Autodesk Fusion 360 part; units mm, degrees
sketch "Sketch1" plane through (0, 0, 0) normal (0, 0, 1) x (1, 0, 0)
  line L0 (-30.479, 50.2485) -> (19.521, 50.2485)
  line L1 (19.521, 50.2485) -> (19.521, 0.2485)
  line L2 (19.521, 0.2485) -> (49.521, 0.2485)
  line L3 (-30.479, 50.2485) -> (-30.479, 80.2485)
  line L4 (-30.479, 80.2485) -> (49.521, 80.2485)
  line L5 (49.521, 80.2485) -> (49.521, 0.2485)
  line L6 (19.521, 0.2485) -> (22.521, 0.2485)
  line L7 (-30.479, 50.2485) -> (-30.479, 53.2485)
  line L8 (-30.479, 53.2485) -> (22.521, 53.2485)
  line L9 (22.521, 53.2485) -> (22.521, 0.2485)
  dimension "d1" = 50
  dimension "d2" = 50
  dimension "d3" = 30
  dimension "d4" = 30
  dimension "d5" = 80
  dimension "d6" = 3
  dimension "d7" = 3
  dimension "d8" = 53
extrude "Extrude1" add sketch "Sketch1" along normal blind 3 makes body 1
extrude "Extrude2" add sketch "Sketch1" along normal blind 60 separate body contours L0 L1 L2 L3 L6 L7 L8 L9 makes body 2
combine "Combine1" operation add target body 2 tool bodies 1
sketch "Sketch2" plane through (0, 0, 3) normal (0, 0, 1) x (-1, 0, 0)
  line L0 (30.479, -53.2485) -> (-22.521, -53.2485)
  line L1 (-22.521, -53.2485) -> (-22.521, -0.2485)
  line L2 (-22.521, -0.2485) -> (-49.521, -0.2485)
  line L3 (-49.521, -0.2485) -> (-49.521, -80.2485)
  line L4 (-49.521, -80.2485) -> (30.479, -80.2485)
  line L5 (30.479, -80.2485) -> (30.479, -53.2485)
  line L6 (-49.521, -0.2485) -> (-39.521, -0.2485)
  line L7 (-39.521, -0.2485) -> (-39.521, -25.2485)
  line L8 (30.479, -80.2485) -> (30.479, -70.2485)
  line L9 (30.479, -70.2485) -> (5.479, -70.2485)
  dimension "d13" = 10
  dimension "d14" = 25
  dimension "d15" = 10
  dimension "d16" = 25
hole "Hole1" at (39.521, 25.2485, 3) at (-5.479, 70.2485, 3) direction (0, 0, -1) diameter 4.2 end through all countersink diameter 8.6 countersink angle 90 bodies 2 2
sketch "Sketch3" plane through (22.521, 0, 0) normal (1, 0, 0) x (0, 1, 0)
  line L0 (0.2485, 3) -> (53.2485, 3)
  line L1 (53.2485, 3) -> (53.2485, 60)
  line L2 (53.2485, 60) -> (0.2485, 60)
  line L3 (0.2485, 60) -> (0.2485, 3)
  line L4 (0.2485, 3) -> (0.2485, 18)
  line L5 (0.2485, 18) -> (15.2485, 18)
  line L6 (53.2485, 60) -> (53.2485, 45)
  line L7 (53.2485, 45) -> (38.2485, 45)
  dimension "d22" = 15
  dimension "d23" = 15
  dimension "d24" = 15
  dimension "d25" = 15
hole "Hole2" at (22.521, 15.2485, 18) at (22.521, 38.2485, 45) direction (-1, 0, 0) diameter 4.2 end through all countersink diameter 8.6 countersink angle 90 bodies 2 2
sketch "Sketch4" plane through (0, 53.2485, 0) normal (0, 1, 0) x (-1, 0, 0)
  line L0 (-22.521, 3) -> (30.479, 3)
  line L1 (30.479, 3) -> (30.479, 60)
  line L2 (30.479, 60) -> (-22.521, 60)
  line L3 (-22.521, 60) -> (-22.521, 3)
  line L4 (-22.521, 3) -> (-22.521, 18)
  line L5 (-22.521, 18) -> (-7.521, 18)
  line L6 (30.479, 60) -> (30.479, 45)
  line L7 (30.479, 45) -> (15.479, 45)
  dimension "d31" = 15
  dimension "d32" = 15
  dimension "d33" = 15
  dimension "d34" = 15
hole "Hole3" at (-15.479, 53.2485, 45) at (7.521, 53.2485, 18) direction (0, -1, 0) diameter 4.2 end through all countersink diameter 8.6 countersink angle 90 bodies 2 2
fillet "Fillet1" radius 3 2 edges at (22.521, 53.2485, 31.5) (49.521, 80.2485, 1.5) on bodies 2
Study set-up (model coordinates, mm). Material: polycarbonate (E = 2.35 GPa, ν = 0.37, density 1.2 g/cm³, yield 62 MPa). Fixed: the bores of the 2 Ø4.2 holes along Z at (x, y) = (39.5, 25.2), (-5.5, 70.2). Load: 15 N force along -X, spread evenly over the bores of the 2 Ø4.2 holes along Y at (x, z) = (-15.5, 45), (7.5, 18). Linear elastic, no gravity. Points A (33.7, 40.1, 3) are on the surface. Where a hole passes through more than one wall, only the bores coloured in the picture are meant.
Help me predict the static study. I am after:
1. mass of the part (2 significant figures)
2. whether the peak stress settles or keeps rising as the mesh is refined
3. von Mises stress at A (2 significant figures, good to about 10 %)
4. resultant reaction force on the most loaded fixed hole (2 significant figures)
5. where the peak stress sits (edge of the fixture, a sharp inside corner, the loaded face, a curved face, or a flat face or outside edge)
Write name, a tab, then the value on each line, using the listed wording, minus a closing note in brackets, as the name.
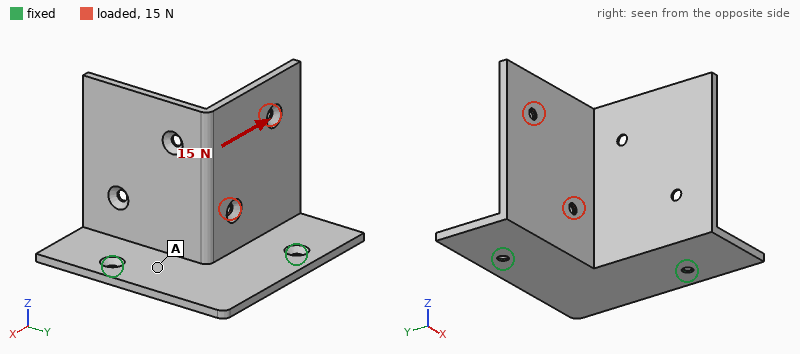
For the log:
mass of the part	34 g
whether the peak stress settles or keeps rising as the mesh is refined	keeps rising
von Mises stress at A	1.2 MPa
resultant reaction force on the most loaded fixed hole	9.9 N
where the peak stress sits	edge of the fixture
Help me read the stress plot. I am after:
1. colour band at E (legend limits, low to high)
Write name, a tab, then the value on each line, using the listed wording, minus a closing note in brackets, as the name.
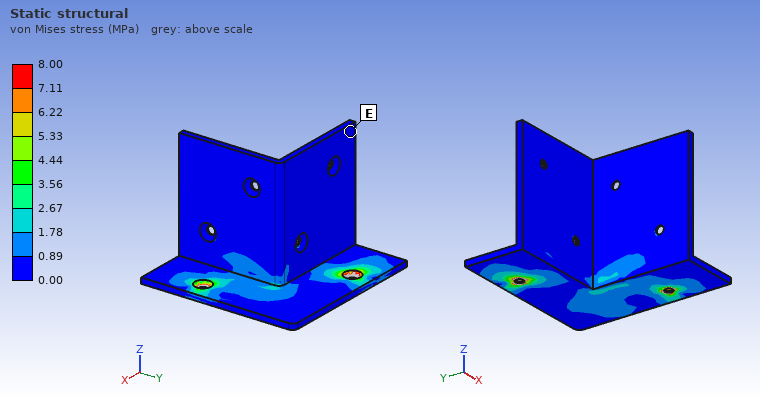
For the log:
colour band at E	0.00 to 0.89 MPa
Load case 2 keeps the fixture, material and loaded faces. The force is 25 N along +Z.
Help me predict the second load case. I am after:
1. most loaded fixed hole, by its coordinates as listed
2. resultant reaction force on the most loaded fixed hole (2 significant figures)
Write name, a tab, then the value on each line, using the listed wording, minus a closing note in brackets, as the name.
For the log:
most loaded fixed hole, by its coordinates as listed	(-5.5, 70.2)
resultant reaction force on the most loaded fixed hole	23 N
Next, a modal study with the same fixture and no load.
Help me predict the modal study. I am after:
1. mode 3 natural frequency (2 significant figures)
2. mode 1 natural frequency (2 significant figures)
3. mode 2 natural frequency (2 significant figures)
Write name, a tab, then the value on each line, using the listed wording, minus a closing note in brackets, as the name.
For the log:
mode 3 natural frequency	330 Hz
mode 1 natural frequency	120 Hz
mode 2 natural frequency	290 Hz
